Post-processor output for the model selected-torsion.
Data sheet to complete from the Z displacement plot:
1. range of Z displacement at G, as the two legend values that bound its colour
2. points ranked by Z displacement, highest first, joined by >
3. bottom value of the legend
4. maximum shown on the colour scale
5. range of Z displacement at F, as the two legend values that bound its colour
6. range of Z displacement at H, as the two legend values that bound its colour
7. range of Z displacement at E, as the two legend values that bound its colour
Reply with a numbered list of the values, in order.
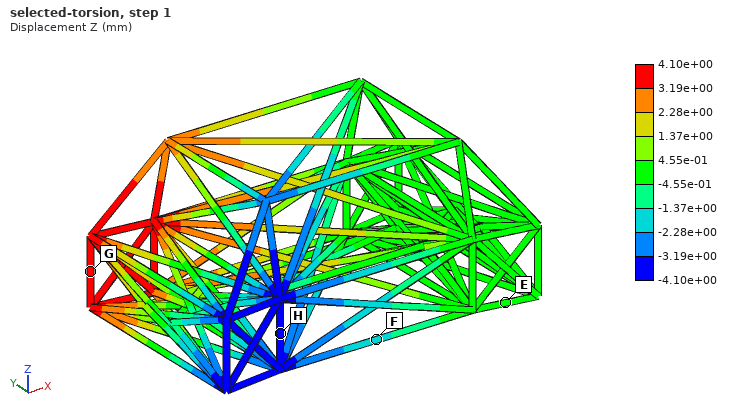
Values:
1. 3.19e+00 to 4.10e+00 mm
2. G > E > F > H
3. -4.10e+00 mm
4. 4.10e+00 mm
5. -2.28e+00 to -1.37e+00 mm
6. -4.10e+00 to -3.19e+00 mm
7. -4.55e-01 to 4.55e-01 mm
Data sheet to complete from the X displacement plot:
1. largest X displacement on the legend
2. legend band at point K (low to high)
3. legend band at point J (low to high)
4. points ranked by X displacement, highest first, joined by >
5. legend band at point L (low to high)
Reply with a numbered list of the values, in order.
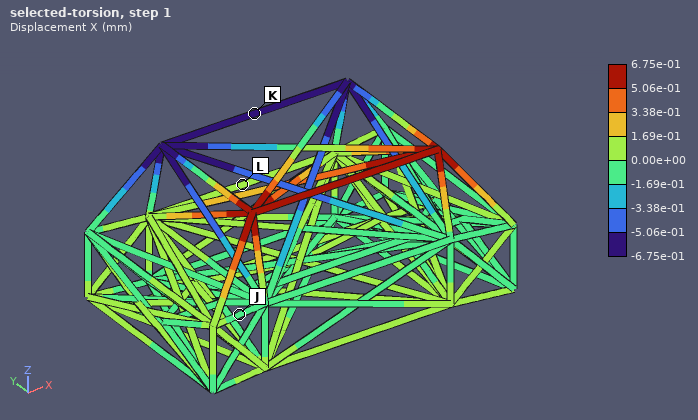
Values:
1. 6.75e-01 mm
2. -6.75e-01 to -5.06e-01 mm
3. -1.69e-01 to 0.00e+00 mm
4. L > J > K
5. 0.00e+00 to 1.69e-01 mm
